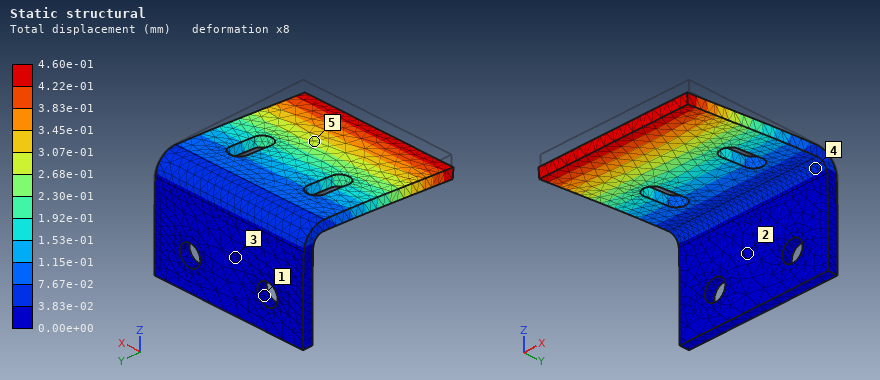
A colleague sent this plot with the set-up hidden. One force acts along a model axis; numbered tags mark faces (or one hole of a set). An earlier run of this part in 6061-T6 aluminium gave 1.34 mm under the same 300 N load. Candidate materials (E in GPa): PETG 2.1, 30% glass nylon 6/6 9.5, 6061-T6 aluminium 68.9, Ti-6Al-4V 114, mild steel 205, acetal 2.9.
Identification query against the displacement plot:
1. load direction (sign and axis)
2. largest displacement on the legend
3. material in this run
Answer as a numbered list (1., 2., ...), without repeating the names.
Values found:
1. -Z
2. 4.60e-01 mm
3. mild steel
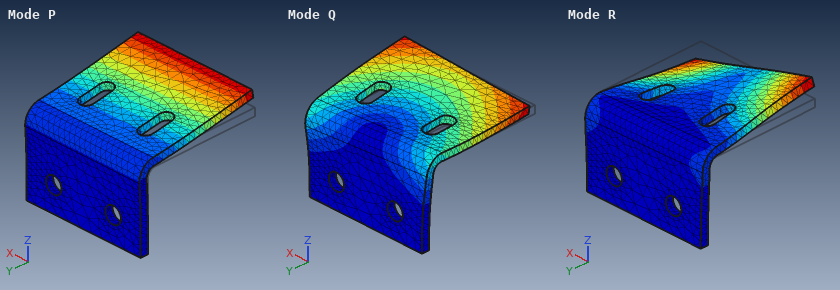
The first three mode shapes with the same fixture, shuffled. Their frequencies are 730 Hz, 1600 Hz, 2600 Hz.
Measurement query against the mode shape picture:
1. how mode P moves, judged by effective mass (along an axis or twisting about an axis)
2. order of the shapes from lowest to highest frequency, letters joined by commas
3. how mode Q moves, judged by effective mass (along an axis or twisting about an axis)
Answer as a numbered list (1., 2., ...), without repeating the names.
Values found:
1. along Z
2. P, Q, R
3. along X
